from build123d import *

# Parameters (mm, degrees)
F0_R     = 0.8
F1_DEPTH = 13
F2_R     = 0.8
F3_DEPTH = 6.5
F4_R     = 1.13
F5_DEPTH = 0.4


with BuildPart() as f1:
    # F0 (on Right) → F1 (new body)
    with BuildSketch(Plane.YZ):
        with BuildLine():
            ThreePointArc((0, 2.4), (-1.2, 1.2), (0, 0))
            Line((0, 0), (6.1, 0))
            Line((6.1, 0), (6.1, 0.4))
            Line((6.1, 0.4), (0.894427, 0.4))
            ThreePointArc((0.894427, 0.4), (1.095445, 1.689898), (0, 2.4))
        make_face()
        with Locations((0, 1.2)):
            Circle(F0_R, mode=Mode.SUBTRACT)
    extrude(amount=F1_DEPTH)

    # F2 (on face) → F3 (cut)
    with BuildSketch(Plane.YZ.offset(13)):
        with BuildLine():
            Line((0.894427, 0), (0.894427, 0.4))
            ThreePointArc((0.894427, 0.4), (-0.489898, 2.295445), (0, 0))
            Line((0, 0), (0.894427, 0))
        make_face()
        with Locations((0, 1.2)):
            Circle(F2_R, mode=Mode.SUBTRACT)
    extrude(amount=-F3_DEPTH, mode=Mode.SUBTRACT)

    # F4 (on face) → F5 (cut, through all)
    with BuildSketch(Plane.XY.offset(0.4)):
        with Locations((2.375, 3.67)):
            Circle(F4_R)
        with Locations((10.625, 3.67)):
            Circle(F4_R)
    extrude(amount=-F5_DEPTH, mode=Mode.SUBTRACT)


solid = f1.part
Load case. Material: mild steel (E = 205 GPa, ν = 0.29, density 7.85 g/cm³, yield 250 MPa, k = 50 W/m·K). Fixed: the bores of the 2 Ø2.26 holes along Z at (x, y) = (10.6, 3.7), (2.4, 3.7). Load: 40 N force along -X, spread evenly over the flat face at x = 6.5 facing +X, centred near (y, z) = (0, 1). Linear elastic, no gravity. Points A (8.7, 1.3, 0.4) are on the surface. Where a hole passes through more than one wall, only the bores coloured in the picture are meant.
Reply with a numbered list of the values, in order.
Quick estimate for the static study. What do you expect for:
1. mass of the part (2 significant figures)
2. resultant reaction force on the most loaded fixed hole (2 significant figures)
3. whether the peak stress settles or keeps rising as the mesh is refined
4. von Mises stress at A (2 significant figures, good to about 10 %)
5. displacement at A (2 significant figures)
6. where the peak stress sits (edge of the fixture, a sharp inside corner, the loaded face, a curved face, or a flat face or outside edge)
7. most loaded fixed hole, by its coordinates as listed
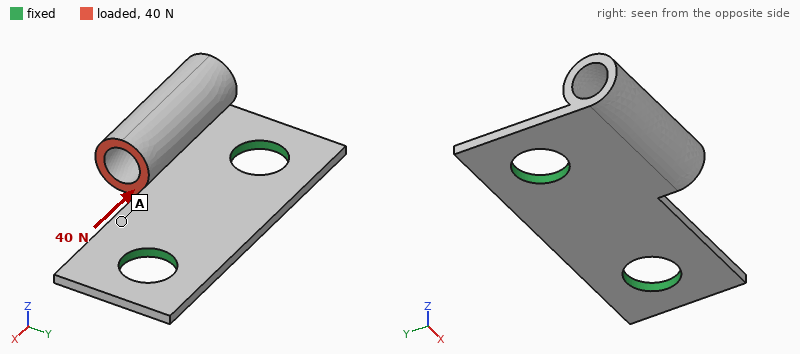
1. 0.32 g
2. 29 N
3. keeps rising
4. 24 MPa
5. 2.8 µm
6. a sharp inside corner
7. (2.4, 3.7)
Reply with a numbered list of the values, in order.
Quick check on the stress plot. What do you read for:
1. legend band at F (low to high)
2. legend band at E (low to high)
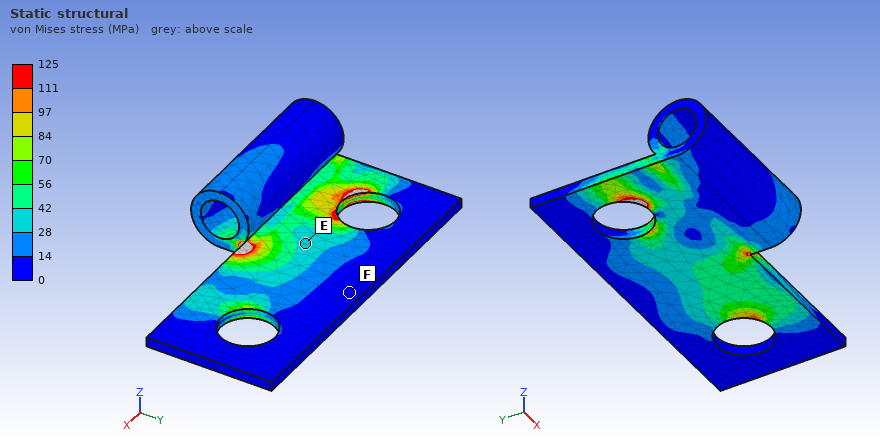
1. 0 to 14 MPa
2. 28 to 42 MPa
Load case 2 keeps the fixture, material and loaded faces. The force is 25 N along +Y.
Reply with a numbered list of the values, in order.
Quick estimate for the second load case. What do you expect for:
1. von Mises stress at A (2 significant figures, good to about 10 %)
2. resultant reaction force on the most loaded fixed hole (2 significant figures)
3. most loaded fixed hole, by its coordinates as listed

1. 41 MPa
2. 15 N
3. (2.4, 3.7)
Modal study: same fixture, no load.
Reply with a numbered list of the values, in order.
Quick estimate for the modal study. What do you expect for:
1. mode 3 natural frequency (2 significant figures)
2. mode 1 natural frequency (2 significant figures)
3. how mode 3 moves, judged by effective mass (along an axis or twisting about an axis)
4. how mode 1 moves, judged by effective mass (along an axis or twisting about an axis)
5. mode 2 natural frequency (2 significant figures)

1. 46 kHz
2. 11 kHz
3. along Z
4. along Z
5. 24 kHz
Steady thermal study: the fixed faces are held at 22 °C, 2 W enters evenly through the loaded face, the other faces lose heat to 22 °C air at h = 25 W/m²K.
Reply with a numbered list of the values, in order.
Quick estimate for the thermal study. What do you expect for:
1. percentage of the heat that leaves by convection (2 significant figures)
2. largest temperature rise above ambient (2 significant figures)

1. 5.3 %
2. 73 K
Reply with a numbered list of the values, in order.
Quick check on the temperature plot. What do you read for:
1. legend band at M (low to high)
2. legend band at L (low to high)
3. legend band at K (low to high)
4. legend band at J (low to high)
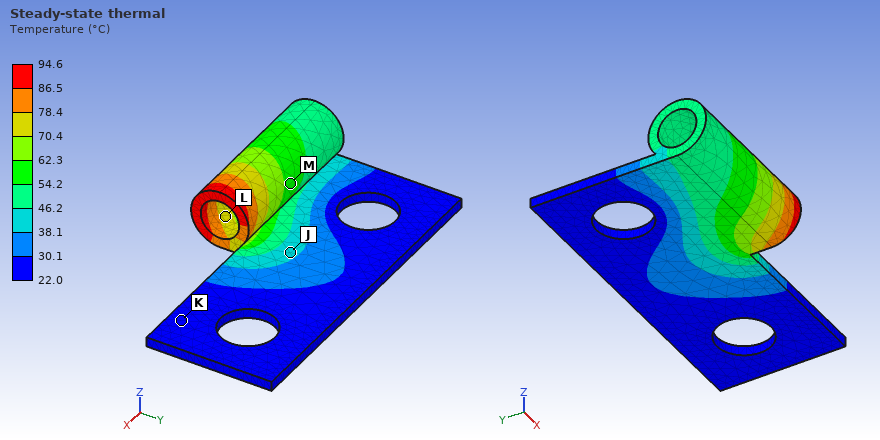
1. 54.2 to 62.3 °C
2. 70.4 to 78.4 °C
3. 22.0 to 30.1 °C
4. 38.1 to 46.2 °C
